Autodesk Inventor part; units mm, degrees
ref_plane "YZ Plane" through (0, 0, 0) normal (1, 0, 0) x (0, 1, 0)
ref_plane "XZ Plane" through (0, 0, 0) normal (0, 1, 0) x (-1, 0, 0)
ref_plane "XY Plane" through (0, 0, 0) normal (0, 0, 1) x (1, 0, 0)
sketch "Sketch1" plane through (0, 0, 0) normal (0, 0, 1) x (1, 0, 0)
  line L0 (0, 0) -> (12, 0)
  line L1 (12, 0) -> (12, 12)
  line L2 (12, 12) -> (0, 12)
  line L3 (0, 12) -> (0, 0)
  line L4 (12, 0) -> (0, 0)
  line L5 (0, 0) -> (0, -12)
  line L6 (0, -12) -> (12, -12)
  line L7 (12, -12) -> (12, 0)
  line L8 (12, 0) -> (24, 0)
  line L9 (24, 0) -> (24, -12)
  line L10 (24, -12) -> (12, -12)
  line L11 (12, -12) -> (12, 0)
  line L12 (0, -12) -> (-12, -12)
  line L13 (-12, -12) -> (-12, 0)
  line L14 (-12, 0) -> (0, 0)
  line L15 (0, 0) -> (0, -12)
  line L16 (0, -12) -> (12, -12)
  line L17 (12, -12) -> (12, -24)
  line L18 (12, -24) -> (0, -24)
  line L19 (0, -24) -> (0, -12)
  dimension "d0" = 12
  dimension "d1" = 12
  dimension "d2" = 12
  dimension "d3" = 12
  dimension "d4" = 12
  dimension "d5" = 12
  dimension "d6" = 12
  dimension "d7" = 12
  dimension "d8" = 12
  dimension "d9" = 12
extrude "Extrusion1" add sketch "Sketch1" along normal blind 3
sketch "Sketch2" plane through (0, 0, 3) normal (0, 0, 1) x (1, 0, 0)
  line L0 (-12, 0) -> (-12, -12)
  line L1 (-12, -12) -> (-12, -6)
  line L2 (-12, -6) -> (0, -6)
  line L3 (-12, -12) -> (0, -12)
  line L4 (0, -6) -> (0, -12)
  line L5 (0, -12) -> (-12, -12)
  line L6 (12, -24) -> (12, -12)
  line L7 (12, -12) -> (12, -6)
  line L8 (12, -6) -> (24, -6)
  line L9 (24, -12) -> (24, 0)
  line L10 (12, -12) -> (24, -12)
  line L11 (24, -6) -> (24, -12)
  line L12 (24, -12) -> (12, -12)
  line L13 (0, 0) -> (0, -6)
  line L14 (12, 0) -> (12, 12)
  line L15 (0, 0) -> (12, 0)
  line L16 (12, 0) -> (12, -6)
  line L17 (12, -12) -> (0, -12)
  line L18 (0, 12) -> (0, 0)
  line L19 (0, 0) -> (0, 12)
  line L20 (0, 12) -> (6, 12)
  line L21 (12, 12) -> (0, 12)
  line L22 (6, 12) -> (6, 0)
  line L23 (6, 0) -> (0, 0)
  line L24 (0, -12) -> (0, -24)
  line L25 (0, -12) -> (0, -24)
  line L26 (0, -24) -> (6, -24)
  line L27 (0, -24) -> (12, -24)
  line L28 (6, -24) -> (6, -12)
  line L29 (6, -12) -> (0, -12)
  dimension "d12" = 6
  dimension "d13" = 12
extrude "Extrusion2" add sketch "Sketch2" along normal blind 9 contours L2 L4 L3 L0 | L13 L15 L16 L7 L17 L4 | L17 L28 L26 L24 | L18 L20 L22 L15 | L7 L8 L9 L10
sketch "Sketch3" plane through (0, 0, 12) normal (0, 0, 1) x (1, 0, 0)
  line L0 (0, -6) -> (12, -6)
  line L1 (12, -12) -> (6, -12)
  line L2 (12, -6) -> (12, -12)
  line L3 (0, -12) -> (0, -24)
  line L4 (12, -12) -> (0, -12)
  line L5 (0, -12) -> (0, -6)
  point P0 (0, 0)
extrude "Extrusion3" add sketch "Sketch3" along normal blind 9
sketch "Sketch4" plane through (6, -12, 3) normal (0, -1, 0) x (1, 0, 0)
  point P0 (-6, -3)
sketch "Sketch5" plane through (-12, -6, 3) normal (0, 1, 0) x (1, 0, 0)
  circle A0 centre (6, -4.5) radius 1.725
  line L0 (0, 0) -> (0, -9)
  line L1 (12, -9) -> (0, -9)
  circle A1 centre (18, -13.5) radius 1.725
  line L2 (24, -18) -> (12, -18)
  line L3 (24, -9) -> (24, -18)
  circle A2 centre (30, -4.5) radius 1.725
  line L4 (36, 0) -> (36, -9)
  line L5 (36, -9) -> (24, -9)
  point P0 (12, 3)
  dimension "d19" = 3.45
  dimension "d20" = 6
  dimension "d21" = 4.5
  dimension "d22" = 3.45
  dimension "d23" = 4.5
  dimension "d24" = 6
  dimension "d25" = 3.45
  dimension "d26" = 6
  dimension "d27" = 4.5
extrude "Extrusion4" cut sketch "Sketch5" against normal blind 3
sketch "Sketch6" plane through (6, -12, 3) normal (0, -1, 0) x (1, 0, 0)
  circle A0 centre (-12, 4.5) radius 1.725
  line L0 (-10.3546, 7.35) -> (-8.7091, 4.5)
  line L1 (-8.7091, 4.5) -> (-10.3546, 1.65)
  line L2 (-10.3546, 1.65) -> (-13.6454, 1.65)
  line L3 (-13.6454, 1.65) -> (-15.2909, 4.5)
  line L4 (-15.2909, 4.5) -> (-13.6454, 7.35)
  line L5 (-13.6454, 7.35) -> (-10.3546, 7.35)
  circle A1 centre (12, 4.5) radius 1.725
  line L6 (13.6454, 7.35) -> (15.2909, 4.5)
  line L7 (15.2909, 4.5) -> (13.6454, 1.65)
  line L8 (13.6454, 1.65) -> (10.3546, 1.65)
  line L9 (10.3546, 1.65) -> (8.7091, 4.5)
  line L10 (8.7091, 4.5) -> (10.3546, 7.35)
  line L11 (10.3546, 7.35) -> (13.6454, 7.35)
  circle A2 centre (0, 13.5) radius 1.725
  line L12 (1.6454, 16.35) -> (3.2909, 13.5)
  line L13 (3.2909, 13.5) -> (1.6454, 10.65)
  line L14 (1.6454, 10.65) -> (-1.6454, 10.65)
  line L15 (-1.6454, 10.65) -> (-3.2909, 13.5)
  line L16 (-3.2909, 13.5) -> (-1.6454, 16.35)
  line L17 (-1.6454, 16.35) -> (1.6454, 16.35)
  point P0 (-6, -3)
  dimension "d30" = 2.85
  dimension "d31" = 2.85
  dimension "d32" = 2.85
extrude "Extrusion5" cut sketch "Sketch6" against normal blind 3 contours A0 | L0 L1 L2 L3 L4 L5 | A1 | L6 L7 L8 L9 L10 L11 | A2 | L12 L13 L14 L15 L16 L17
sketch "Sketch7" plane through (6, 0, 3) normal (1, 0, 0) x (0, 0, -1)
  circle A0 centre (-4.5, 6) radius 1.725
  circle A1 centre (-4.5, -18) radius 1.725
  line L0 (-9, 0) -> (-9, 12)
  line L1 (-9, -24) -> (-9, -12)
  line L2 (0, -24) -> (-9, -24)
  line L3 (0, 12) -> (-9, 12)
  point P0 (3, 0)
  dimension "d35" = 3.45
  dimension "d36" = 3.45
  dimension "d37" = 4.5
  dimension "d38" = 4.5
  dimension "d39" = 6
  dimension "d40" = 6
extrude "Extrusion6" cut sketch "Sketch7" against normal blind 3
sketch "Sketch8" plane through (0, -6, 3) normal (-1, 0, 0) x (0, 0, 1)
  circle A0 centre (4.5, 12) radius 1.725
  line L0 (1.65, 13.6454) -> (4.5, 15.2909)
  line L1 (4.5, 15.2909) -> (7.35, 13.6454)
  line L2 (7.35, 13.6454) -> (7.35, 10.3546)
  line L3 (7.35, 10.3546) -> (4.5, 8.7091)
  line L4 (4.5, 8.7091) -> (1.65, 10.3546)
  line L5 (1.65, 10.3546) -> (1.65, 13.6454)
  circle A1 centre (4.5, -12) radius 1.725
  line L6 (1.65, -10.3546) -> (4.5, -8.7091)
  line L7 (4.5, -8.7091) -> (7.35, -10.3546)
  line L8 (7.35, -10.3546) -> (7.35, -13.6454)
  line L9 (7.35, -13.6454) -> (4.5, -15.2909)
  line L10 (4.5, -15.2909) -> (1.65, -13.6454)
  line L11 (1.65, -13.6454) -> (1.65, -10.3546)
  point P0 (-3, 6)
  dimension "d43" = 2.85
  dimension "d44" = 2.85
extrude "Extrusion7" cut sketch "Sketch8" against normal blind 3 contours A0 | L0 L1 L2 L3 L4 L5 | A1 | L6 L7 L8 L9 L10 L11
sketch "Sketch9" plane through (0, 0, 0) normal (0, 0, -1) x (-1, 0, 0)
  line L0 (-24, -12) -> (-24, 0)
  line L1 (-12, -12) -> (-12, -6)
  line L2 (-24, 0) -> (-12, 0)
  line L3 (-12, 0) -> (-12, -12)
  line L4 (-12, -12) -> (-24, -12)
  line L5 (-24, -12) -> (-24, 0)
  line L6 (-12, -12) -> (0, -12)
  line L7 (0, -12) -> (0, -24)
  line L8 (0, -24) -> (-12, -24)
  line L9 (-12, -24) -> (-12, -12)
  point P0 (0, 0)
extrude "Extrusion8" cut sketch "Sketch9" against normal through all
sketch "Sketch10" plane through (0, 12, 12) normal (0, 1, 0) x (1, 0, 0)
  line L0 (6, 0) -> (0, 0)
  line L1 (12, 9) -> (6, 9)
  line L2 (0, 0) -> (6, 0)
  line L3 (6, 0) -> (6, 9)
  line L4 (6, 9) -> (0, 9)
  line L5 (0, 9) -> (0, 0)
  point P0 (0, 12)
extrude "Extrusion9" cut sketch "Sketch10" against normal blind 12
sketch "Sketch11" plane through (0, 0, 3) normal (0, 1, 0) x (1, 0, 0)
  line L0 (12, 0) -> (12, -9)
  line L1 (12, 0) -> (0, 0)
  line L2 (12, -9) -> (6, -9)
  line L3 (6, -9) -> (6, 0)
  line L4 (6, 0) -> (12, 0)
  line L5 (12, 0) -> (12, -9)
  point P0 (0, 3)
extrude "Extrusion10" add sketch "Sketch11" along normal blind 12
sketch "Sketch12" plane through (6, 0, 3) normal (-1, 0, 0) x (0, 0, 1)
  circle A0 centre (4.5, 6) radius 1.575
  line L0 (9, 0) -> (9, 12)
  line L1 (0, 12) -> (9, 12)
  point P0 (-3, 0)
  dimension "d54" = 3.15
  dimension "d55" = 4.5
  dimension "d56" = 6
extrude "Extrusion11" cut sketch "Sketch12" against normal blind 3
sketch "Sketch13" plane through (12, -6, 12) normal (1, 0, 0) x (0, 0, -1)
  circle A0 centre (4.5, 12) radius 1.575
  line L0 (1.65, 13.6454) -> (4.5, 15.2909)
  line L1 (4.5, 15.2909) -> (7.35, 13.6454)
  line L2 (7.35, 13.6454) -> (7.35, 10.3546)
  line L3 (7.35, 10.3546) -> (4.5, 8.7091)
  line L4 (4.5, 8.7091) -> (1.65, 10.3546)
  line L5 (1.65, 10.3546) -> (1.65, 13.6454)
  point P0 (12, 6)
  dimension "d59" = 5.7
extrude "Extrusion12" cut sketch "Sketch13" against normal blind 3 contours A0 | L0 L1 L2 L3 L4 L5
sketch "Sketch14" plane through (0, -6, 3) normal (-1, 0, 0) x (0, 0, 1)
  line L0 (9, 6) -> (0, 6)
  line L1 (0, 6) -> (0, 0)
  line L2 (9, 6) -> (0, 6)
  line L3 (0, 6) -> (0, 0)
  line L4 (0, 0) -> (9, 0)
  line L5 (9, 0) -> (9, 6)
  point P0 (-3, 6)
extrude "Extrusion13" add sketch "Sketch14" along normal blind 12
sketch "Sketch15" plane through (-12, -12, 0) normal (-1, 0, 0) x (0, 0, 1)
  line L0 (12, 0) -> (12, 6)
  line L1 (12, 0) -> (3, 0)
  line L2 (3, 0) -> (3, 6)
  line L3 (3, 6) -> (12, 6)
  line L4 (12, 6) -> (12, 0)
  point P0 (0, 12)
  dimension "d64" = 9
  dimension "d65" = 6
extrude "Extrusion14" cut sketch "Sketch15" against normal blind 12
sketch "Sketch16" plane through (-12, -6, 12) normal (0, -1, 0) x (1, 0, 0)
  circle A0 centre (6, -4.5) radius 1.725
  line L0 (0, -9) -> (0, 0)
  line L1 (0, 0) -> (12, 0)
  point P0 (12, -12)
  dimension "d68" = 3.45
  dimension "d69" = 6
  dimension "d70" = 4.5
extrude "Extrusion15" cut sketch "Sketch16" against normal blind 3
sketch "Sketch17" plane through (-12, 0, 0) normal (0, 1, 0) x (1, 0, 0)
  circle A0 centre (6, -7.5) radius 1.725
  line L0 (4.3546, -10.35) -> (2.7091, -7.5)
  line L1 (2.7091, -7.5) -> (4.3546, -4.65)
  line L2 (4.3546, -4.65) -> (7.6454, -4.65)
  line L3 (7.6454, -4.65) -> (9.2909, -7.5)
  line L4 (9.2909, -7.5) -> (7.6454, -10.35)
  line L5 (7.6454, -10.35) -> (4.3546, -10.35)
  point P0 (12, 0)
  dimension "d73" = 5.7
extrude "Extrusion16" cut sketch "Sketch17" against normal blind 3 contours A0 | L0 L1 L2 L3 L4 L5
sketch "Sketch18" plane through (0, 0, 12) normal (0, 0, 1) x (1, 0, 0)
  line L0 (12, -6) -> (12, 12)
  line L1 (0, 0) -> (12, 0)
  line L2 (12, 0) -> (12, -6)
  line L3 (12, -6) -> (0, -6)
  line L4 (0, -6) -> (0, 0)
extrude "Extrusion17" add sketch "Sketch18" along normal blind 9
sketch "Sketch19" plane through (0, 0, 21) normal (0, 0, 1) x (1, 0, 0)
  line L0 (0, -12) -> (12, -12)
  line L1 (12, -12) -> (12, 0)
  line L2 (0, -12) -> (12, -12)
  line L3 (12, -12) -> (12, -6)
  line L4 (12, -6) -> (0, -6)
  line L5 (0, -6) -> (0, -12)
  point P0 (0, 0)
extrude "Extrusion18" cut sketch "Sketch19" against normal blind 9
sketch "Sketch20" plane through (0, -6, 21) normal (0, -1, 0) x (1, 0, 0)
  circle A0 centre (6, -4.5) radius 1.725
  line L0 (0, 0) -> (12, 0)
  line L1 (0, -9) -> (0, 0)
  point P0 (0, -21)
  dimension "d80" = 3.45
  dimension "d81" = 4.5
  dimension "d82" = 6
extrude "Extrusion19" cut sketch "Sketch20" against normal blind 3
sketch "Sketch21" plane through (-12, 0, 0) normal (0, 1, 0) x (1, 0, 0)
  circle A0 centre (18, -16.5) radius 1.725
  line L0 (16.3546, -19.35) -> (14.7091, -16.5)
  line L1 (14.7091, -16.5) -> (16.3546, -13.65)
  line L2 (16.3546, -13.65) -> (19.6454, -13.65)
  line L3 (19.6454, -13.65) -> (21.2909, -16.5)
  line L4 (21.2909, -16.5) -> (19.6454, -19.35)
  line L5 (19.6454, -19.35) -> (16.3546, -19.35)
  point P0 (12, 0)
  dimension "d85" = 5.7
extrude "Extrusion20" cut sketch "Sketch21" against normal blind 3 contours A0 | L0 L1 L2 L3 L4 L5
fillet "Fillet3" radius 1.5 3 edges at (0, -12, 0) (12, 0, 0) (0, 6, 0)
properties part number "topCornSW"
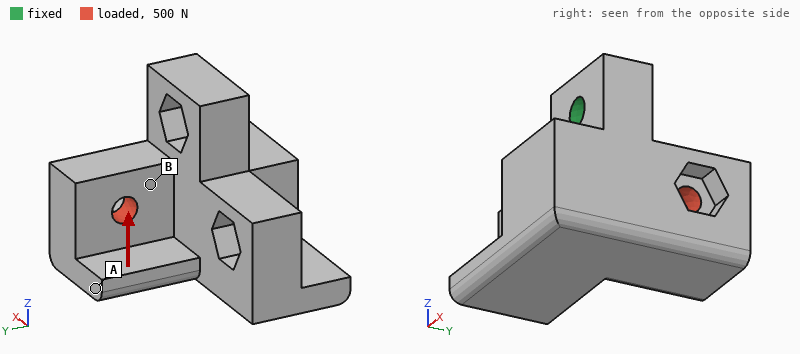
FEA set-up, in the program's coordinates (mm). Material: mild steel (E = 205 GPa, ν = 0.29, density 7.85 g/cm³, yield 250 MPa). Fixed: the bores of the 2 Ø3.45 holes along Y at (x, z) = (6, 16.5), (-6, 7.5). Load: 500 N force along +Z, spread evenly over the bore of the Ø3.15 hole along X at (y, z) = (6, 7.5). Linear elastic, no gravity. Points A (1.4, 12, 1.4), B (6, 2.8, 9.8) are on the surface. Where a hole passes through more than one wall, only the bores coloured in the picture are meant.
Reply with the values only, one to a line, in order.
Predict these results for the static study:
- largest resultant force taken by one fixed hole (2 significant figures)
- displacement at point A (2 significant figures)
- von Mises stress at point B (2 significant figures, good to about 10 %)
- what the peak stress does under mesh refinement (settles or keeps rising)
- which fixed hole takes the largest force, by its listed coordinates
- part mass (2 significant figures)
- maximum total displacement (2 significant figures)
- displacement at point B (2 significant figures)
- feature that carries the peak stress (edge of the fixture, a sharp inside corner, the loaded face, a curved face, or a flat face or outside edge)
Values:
520 N
15 µm
27 MPa
keeps rising
(6, 16.5)
33 g
17 µm
6.0 µm
edge of the fixture
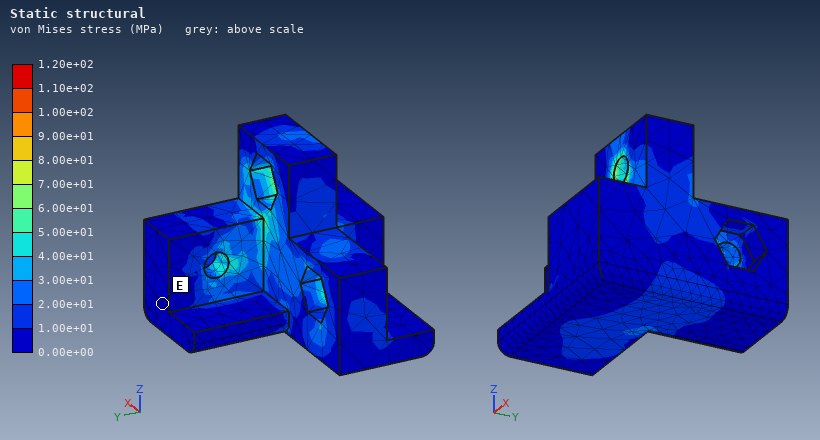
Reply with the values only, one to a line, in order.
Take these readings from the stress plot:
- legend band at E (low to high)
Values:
0.00e+00 to 1.00e+01 MPa
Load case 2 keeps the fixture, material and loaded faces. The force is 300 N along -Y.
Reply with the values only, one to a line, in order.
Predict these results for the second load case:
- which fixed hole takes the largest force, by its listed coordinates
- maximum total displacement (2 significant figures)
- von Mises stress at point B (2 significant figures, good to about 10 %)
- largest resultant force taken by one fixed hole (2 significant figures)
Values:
(6, 16.5)
6.6 µm
11 MPa
210 N
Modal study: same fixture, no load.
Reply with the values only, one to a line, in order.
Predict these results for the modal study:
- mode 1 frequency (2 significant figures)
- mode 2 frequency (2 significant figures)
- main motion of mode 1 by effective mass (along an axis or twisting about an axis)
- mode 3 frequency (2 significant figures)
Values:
7600 Hz
19 kHz
along Y
27 kHz
